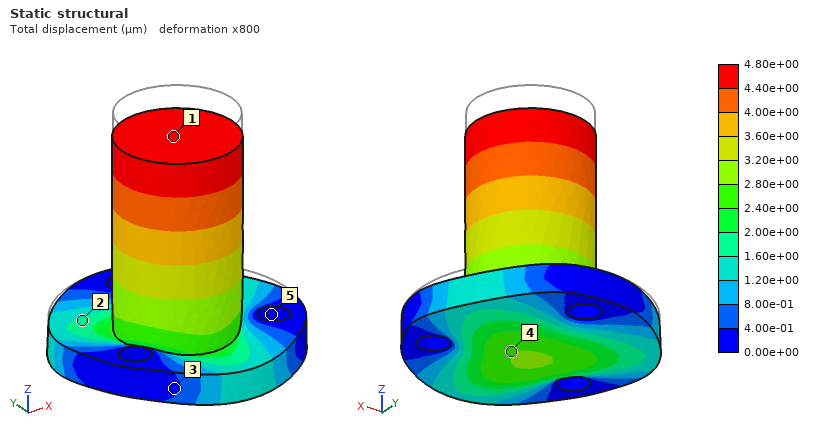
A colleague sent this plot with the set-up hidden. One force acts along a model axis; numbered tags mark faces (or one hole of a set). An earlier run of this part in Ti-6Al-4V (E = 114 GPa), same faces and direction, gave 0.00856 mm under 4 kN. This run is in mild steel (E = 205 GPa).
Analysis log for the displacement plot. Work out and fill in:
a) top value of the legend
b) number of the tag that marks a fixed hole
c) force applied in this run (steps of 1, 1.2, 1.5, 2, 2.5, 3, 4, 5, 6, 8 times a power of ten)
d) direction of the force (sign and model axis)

4.80e+00 µm
5
4 kN
-Z
